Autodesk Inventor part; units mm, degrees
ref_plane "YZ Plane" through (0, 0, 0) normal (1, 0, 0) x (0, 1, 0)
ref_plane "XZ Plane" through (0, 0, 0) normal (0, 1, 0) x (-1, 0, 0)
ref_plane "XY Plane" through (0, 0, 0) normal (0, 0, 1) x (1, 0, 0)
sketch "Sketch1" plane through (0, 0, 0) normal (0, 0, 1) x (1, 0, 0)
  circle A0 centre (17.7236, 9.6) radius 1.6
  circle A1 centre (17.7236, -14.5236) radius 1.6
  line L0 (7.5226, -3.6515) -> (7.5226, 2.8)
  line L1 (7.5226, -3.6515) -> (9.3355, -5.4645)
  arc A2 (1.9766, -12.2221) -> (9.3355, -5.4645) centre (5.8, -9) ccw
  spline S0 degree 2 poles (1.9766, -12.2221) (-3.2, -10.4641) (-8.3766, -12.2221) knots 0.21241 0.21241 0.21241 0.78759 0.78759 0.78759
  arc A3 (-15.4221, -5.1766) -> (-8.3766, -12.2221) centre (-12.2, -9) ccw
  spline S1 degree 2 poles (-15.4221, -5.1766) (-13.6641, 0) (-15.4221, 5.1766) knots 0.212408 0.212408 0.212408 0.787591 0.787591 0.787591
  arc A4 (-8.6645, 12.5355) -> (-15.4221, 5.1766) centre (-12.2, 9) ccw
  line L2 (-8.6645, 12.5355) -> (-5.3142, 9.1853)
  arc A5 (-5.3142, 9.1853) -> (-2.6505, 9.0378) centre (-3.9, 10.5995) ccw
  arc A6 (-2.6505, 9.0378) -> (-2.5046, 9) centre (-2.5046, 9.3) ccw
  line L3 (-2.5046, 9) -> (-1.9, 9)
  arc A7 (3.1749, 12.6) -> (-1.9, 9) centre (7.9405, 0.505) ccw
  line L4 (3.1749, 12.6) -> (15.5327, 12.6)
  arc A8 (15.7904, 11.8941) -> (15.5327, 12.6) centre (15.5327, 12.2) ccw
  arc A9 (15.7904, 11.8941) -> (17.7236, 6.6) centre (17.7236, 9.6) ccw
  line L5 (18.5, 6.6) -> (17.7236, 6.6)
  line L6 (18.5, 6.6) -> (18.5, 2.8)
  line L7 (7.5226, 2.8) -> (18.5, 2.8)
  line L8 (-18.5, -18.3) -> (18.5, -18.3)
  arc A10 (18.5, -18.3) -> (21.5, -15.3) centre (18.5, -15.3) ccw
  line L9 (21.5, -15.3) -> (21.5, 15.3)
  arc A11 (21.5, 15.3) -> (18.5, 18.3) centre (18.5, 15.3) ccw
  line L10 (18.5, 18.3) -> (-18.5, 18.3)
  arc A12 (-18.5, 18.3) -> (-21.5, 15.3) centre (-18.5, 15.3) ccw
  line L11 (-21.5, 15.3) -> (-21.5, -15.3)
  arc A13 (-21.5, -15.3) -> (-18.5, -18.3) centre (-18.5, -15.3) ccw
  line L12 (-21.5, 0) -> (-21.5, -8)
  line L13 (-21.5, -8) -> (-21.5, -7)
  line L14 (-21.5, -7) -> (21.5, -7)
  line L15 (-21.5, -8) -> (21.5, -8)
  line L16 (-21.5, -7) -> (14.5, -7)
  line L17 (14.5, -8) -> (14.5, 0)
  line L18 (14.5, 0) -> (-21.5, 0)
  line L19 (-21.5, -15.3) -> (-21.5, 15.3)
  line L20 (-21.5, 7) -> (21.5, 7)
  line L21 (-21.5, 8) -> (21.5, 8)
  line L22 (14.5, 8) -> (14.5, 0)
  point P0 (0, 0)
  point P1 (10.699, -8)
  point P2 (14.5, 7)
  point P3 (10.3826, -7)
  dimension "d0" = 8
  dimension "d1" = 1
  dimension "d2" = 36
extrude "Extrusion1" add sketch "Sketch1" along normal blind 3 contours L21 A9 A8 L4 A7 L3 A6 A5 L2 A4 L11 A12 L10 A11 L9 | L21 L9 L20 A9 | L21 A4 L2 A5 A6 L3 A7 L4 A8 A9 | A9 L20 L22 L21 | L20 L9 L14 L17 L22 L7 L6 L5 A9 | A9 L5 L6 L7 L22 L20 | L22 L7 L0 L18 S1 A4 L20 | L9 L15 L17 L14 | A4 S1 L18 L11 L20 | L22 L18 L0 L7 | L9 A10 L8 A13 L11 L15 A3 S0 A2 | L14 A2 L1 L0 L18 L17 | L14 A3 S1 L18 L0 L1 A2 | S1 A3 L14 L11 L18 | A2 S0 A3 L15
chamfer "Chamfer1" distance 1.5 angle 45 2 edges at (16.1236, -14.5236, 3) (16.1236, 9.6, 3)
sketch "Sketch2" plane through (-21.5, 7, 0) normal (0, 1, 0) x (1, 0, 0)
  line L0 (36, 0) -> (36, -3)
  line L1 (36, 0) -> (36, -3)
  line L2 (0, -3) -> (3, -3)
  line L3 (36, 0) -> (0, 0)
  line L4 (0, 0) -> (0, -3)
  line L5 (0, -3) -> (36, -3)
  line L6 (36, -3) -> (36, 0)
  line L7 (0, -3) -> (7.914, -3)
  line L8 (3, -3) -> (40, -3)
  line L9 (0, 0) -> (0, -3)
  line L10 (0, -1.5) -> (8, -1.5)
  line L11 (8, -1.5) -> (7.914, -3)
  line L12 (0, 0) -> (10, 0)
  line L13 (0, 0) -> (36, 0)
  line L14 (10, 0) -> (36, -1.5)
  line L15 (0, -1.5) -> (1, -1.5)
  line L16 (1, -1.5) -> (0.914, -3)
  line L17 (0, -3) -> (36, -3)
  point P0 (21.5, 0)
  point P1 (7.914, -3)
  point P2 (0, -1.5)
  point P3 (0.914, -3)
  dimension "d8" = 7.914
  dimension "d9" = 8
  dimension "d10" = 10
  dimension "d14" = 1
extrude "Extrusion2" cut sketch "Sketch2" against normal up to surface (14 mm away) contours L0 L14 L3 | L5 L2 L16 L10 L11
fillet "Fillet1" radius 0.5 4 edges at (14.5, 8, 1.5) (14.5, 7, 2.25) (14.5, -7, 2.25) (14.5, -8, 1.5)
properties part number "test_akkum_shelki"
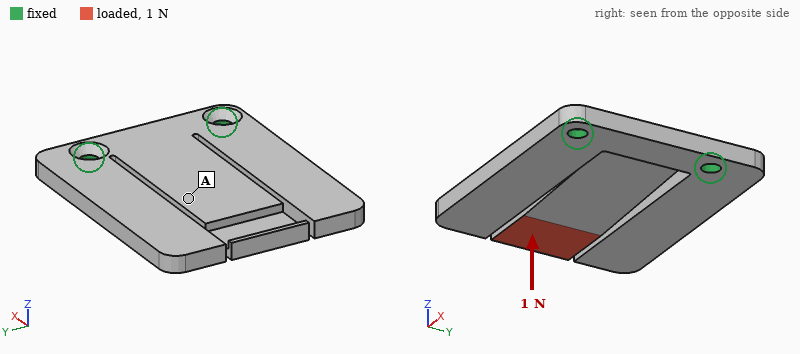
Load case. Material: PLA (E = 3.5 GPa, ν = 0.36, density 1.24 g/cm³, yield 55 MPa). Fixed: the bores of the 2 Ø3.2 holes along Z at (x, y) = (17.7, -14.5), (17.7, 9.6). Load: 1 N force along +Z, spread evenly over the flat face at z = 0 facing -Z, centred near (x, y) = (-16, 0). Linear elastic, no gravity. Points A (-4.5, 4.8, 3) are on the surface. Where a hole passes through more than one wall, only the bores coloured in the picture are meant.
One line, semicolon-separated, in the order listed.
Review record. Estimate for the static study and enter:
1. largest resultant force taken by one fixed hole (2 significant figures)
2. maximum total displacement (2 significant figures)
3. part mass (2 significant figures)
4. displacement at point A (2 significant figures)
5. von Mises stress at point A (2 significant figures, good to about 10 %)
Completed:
1.2 N; 0.60 mm; 4.9 g; 0.27 mm; 0.79 MPa
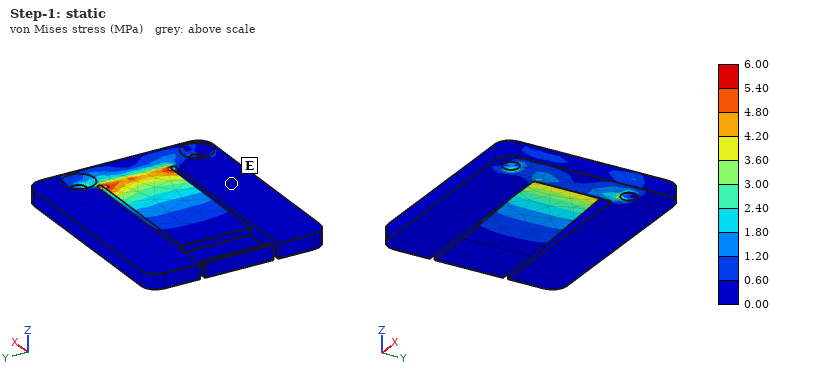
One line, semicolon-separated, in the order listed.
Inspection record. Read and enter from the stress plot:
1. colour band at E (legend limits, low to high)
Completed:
0.00 to 0.60 MPa
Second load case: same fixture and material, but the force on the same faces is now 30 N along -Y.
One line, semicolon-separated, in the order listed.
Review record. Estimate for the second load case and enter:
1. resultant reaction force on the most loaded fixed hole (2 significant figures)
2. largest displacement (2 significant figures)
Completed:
54 N; 0.51 mm
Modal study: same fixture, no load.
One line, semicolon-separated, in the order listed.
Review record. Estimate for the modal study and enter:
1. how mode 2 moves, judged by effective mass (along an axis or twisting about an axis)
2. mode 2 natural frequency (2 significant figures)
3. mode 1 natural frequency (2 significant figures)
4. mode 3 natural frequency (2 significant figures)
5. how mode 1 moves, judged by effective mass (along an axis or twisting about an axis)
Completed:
along Z; 470 Hz; 300 Hz; 500 Hz; along Z
